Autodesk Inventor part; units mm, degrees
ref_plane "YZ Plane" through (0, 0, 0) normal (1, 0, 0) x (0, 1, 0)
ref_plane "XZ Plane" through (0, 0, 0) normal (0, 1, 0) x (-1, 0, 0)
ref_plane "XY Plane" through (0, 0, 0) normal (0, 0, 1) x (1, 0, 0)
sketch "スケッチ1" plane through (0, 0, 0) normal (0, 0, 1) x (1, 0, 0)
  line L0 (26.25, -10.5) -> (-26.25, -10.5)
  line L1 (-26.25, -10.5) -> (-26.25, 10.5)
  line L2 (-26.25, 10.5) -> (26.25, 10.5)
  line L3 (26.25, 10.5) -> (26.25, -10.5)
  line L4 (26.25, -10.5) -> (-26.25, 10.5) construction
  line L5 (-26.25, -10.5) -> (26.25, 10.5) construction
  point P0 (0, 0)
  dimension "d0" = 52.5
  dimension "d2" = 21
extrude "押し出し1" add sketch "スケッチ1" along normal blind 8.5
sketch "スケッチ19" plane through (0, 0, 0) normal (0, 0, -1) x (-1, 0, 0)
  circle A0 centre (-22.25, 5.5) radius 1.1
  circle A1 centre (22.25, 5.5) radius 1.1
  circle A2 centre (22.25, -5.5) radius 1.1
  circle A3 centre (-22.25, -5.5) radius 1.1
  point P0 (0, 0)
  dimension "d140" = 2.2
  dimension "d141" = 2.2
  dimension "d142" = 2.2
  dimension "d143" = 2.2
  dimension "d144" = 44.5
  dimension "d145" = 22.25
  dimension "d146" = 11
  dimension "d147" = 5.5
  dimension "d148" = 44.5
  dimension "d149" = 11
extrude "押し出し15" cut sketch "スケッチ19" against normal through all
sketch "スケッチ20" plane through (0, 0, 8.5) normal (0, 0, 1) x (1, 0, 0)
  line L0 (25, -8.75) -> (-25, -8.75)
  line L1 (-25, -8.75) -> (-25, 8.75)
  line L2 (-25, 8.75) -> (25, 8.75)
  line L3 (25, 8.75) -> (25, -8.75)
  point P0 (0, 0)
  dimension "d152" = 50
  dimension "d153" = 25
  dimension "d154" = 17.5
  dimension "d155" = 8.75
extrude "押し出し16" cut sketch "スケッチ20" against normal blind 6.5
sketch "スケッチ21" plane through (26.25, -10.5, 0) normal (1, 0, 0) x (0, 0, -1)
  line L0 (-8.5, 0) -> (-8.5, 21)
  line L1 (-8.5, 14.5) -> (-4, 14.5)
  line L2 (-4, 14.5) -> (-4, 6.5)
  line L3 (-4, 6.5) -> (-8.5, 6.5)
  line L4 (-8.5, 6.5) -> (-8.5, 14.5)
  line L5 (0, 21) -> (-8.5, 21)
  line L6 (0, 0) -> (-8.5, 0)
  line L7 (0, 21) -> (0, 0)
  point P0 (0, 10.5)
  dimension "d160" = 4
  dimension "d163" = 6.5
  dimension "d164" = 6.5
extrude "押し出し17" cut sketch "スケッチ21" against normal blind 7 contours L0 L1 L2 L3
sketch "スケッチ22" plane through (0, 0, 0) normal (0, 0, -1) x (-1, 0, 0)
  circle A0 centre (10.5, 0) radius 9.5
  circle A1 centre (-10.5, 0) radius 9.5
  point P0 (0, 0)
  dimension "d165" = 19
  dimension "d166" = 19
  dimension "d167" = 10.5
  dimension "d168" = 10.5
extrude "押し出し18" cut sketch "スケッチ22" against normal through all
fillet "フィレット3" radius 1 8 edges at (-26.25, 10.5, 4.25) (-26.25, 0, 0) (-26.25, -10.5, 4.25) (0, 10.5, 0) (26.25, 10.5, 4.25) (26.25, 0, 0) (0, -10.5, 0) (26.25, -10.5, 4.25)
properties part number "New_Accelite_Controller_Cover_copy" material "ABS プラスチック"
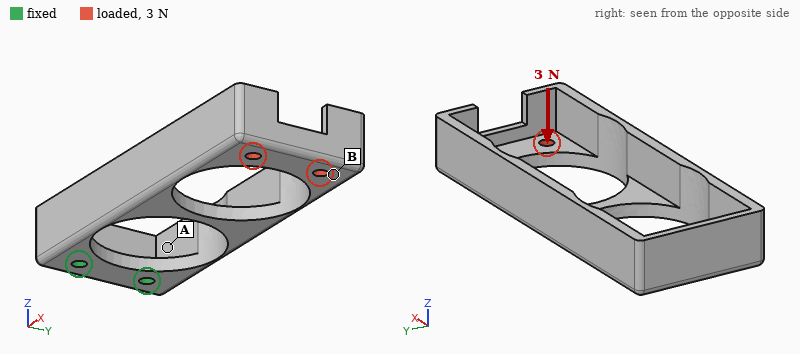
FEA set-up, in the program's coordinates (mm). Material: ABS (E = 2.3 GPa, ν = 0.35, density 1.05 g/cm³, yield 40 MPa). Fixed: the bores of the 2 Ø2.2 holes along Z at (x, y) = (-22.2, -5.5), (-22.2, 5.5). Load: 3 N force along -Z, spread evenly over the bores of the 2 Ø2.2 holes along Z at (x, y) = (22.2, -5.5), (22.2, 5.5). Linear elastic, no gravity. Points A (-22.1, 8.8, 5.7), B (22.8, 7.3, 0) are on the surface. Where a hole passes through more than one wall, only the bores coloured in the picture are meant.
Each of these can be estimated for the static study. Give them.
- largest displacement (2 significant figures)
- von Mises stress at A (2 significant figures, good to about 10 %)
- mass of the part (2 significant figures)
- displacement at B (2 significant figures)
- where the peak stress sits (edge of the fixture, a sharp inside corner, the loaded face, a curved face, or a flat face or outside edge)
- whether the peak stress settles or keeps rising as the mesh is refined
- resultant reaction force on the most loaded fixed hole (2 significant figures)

0.68 mm
2.4 MPa
2.5 g
0.62 mm
edge of the fixture
keeps rising
1.5 N
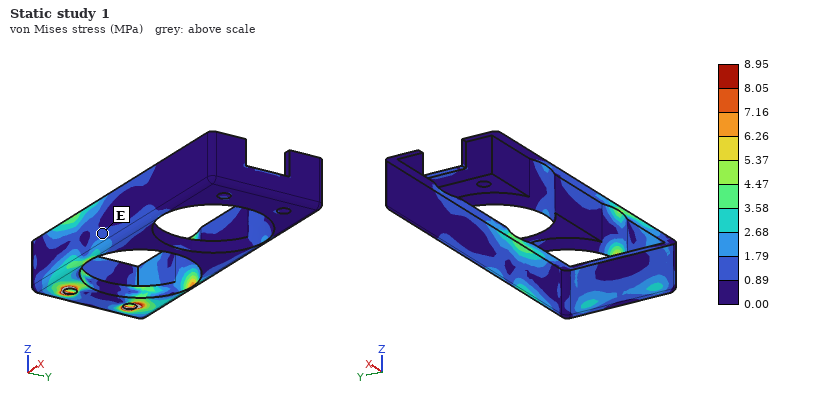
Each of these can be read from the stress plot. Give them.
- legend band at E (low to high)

0.89 to 1.79 MPa
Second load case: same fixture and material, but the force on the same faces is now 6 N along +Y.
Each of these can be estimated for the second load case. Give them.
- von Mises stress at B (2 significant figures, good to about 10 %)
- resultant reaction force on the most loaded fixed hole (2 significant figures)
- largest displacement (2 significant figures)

1.2 MPa
18 N
0.47 mm
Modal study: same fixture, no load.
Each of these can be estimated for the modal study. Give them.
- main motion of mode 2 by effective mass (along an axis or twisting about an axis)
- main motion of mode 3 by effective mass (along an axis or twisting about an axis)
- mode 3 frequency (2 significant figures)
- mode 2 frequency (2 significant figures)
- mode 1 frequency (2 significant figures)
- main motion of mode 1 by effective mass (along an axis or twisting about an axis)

along Y
along Y
700 Hz
530 Hz
370 Hz
along Z
